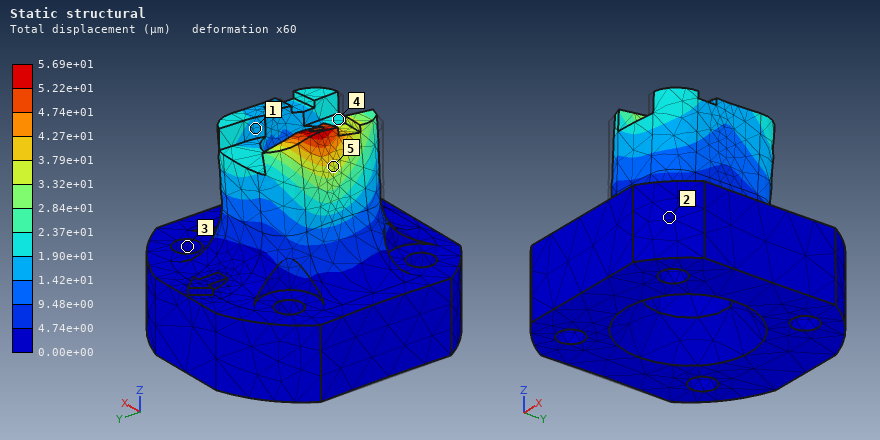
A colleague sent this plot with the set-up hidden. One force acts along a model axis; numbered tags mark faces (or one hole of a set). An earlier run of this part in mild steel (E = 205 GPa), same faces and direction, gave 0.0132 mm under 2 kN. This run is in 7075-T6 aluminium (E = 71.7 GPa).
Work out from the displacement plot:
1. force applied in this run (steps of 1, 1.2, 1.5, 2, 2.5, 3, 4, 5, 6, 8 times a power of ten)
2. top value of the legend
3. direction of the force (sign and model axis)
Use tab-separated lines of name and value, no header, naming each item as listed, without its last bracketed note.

force applied in this run	3 kN
top value of the legend	5.69e+01 µm
direction of the force	+X
